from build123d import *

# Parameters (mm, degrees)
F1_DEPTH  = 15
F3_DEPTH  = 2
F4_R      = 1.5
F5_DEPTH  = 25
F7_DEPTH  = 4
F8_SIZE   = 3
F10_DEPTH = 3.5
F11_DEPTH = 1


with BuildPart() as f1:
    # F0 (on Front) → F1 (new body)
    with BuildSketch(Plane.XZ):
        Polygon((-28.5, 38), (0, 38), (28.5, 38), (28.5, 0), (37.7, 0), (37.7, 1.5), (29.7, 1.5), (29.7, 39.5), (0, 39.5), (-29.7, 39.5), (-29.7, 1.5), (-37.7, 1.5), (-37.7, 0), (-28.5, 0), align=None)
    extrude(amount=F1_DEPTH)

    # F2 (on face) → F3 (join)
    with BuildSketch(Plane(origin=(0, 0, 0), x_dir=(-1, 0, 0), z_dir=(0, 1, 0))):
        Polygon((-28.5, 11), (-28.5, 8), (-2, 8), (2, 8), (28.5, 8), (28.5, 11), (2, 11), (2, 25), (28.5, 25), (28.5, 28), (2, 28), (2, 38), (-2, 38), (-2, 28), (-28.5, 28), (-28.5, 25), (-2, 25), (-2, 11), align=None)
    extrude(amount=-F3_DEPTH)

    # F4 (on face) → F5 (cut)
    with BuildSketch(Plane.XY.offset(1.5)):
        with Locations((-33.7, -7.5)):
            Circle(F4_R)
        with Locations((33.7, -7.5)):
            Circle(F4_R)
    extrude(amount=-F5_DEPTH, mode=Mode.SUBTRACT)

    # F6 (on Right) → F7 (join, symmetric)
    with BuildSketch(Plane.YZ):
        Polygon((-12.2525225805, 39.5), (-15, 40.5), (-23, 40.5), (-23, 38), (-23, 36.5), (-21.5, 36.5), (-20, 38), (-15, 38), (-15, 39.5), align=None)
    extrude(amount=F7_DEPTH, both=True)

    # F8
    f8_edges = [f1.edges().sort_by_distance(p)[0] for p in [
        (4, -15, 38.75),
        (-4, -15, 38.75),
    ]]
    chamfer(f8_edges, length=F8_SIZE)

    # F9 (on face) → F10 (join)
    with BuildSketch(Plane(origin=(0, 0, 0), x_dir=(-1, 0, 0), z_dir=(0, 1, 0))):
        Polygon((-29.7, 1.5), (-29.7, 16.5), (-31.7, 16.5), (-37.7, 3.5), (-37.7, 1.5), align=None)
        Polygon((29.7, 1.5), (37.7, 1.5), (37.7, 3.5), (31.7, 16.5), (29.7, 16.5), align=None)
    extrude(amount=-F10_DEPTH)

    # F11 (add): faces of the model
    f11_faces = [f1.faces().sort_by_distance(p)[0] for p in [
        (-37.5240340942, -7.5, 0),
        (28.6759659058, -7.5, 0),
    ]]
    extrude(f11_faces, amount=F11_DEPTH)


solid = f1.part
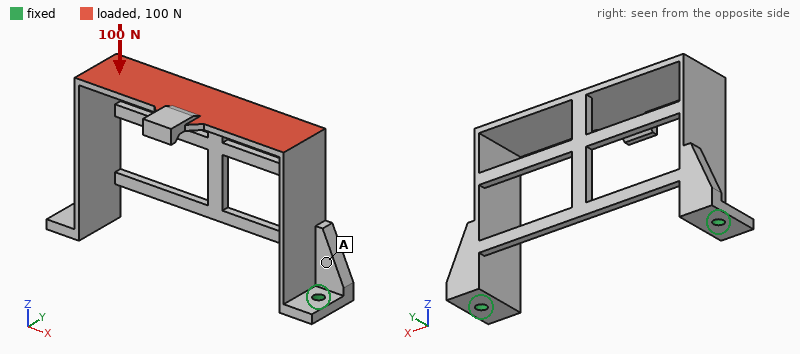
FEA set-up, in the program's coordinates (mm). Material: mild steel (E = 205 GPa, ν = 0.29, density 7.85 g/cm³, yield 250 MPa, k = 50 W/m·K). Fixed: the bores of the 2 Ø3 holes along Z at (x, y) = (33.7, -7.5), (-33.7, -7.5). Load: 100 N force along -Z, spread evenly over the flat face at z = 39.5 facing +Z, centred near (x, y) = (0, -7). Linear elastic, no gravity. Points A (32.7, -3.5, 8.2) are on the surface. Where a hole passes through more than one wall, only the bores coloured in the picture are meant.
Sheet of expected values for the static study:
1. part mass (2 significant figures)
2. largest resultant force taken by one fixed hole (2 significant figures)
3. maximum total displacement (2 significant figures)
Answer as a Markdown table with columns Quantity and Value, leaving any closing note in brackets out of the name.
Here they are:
| Quantity | Value |
|---|---|
| part mass | 39 g |
| largest resultant force taken by one fixed hole | 52 N |
| maximum total displacement | 53 µm |
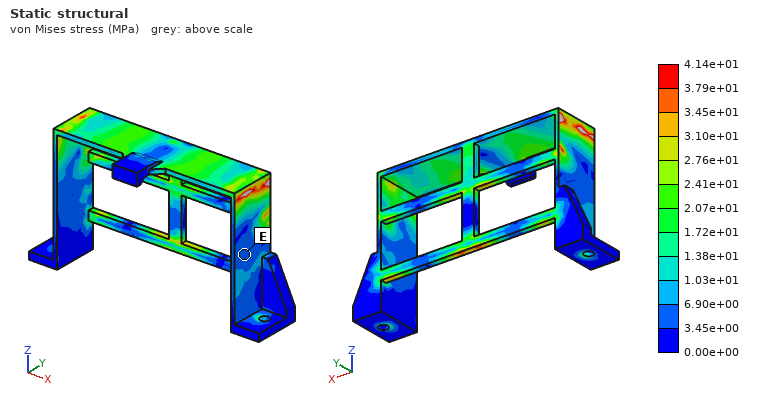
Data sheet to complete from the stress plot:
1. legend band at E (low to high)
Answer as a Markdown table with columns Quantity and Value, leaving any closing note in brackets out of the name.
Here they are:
| Quantity | Value |
|---|---|
| legend band at E | 3.45e+00 to 6.90e+00 MPa |
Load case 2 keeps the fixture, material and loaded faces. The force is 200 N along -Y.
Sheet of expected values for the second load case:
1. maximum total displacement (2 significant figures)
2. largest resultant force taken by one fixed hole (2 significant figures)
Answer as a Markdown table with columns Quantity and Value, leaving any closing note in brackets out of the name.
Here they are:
| Quantity | Value |
|---|---|
| maximum total displacement | 0.13 mm |
| largest resultant force taken by one fixed hole | 140 N |
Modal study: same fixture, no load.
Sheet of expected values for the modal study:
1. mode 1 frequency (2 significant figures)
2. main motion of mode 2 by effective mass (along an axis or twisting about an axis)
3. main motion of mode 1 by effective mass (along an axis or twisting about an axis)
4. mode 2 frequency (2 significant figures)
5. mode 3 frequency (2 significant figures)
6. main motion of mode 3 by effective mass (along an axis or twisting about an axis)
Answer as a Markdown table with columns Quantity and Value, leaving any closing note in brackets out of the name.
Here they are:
| Quantity | Value |
|---|---|
| mode 1 frequency | 1600 Hz |
| main motion of mode 2 by effective mass | along X |
| main motion of mode 1 by effective mass | along Y |
| mode 2 frequency | 1700 Hz |
| mode 3 frequency | 2000 Hz |
| main motion of mode 3 by effective mass | along Z |
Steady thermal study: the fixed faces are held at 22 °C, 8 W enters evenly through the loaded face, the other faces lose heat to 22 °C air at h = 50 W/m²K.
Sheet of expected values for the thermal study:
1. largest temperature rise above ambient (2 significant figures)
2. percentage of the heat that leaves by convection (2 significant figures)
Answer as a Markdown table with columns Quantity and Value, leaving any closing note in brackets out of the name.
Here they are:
| Quantity | Value |
|---|---|
| largest temperature rise above ambient | 56 K |
| percentage of the heat that leaves by convection | 81 % |
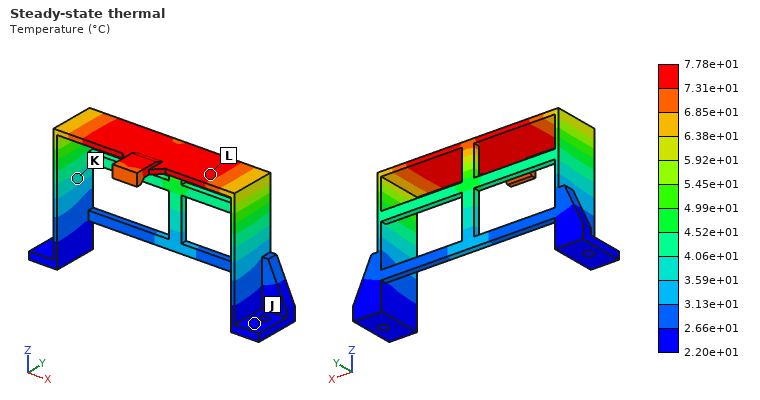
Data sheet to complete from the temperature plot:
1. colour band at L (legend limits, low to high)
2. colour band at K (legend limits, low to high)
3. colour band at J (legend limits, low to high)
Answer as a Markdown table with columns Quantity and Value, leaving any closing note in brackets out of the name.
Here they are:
| Quantity | Value |
|---|---|
| colour band at L | 7.31e+01 to 7.78e+01 °C |
| colour band at K | 3.59e+01 to 4.06e+01 °C |
| colour band at J | 2.20e+01 to 2.66e+01 °C |
